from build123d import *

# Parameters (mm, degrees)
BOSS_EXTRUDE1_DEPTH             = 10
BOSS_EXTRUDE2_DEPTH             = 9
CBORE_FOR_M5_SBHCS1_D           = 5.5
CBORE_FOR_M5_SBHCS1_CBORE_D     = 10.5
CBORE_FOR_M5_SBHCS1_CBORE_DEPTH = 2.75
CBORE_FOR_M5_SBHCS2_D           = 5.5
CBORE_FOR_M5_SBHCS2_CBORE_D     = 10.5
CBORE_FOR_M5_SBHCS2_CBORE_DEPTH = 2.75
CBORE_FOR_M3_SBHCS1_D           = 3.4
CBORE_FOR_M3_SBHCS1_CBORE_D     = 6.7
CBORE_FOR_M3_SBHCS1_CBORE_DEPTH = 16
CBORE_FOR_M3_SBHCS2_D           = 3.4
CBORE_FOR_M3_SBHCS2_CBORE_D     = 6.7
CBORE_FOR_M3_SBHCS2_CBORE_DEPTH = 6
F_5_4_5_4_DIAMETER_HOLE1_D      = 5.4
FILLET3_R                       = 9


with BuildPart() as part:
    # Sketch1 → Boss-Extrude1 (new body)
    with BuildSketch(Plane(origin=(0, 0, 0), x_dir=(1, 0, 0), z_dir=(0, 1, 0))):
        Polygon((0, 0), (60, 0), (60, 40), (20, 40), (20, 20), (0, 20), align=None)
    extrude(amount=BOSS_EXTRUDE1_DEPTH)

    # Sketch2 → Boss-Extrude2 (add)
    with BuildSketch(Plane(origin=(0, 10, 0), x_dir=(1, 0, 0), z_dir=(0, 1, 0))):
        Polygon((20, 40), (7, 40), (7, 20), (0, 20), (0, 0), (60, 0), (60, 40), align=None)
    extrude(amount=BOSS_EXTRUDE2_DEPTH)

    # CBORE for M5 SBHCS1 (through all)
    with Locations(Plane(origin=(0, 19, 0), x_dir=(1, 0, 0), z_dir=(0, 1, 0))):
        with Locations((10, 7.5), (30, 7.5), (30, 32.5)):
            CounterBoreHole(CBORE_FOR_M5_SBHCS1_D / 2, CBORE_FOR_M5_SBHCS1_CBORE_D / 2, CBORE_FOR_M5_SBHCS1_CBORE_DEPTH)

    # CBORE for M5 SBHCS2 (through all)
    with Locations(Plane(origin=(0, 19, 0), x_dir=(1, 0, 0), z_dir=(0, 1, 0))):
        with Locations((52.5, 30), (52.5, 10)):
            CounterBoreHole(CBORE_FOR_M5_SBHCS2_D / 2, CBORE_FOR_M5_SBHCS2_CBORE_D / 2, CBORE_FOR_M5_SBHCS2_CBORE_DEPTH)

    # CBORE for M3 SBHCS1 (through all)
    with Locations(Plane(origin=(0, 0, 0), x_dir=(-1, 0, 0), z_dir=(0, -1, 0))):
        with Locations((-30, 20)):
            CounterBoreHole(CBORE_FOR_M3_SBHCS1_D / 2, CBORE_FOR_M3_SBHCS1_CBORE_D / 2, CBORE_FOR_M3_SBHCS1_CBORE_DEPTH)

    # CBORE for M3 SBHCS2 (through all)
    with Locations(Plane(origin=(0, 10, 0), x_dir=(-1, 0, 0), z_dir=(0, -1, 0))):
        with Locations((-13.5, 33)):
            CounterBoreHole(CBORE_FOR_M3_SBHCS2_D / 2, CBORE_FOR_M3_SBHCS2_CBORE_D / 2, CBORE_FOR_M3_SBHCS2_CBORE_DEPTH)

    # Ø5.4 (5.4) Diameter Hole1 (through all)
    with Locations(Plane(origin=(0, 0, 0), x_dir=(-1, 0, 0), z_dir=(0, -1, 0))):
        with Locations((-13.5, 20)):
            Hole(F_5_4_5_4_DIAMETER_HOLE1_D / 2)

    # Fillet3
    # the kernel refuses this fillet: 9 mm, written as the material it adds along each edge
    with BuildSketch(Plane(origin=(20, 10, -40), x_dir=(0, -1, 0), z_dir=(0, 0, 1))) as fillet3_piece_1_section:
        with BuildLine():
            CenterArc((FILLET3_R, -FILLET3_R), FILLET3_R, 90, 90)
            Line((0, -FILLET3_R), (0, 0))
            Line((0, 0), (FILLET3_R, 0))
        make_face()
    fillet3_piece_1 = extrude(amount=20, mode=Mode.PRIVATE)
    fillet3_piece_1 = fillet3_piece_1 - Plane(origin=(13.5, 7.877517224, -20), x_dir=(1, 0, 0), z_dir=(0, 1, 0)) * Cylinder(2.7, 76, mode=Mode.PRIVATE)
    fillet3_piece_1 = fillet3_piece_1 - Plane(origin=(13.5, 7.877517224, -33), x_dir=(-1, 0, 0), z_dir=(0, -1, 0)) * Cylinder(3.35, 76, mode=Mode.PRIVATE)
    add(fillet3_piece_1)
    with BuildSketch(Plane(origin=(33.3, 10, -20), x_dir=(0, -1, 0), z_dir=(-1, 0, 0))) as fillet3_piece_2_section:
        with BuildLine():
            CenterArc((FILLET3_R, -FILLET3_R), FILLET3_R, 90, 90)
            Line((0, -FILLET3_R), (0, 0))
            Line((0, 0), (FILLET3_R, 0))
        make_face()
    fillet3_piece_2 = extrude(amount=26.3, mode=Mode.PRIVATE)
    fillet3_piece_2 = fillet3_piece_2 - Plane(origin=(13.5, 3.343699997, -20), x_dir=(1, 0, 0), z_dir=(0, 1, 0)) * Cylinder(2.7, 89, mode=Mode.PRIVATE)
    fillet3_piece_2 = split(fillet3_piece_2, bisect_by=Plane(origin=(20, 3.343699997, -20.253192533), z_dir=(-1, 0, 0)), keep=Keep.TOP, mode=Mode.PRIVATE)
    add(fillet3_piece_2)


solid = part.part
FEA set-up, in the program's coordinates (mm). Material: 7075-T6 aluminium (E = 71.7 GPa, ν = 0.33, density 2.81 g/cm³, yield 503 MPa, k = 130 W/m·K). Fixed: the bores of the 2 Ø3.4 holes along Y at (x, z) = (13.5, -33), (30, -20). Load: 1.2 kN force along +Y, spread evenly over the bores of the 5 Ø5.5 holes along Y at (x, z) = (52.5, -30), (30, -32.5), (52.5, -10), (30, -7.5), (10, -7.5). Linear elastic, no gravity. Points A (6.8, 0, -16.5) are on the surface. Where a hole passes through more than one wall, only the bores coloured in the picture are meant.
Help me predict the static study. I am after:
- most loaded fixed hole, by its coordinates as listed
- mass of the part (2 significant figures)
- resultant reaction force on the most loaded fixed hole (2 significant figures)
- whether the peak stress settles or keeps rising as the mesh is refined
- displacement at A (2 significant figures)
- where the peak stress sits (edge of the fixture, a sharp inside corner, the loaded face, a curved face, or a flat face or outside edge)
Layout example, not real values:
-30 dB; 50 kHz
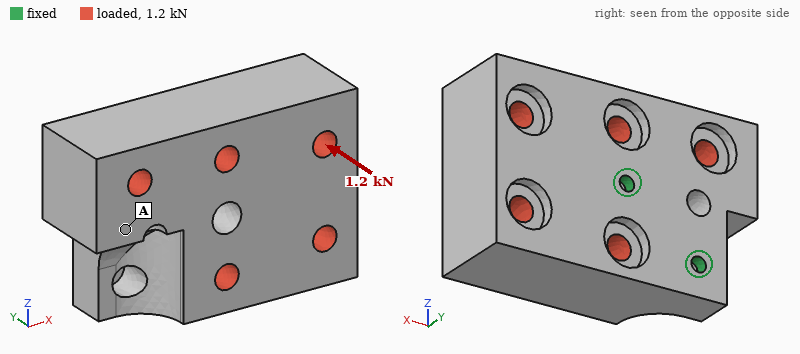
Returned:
(30, -20); 100 g; 1.5 kN; keeps rising; 9.1 µm; edge of the fixture
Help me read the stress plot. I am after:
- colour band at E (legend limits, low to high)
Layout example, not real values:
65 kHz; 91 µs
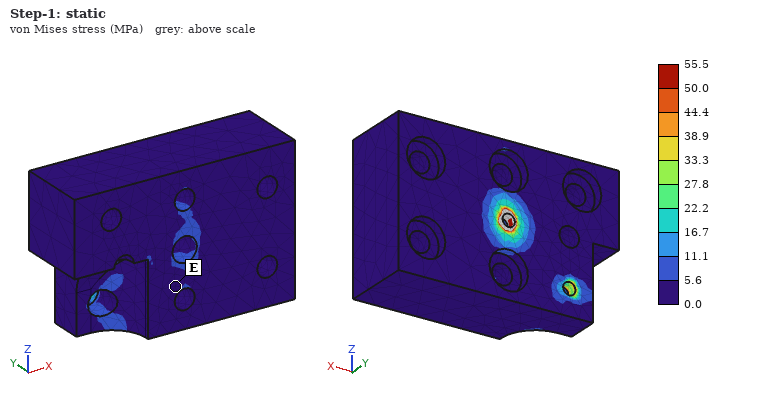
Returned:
0.0 to 5.6 MPa
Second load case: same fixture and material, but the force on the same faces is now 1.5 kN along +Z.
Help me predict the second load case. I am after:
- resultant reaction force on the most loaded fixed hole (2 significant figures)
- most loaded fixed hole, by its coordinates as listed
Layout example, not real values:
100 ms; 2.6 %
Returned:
1.6 kN; (30, -20)
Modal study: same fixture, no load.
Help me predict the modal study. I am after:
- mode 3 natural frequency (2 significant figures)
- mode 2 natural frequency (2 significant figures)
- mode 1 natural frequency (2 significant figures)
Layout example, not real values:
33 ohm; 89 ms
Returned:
6200 Hz; 5200 Hz; 1800 Hz
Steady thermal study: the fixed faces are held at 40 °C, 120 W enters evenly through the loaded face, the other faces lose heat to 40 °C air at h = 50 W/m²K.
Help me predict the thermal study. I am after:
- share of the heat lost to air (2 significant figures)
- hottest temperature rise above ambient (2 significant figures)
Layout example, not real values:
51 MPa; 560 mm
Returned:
15 %; 50 K
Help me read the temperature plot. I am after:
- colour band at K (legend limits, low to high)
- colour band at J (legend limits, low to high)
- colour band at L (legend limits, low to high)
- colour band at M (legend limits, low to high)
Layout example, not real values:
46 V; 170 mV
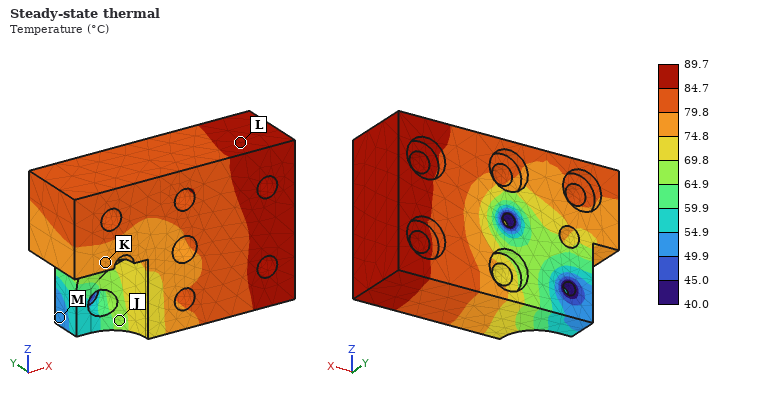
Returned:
74.8 to 79.8 °C; 64.9 to 69.8 °C; 84.7 to 89.7 °C; 49.9 to 54.9 °C
